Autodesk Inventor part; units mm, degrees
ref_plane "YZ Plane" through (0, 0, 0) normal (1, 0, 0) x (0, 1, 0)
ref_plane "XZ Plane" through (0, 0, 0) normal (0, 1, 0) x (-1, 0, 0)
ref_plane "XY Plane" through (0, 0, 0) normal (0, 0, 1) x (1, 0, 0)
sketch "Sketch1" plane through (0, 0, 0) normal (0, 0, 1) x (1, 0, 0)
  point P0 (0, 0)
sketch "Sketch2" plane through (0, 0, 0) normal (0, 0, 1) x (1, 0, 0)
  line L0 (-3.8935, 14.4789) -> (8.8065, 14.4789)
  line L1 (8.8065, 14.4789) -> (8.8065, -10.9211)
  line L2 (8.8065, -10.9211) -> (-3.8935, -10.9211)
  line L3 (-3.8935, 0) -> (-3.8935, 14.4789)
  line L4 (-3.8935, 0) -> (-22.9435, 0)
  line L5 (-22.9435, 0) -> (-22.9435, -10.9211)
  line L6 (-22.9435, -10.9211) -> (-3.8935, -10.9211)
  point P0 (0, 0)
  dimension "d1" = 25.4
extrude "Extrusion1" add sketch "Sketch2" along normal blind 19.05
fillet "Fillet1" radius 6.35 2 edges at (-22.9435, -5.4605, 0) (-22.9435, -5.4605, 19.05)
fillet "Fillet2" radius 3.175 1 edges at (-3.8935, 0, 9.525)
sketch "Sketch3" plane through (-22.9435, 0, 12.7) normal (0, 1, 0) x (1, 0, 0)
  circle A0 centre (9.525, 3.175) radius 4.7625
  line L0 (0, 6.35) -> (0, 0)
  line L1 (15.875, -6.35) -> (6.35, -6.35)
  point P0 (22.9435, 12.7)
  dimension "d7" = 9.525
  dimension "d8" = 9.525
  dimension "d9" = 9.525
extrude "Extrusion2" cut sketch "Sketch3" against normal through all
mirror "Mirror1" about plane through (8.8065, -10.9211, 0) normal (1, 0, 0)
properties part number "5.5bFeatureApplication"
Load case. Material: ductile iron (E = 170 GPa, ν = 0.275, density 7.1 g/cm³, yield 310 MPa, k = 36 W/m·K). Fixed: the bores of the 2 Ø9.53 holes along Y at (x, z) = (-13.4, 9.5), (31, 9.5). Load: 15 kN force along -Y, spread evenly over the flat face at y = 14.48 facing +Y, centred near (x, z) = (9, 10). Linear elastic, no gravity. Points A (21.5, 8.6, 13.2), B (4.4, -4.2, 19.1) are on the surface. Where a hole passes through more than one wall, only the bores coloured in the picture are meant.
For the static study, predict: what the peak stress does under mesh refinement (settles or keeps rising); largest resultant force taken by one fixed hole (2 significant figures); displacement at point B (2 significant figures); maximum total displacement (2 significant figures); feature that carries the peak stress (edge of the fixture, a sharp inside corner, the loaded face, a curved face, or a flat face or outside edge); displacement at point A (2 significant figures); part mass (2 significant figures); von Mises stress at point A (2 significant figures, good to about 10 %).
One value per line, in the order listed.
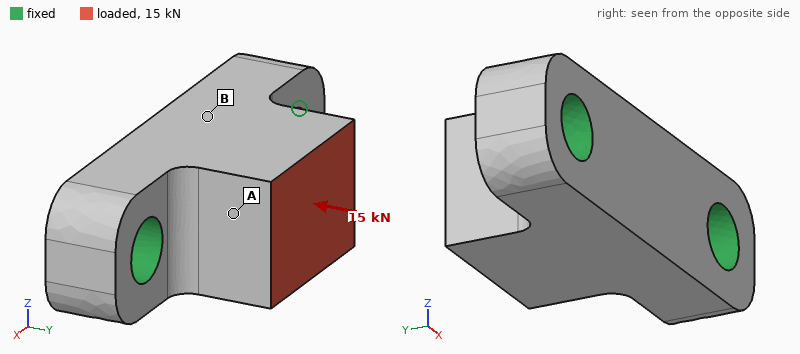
keeps rising
8.0 kN
8.9 µm
11 µm
edge of the fixture
9.4 µm
130 g
37 MPa
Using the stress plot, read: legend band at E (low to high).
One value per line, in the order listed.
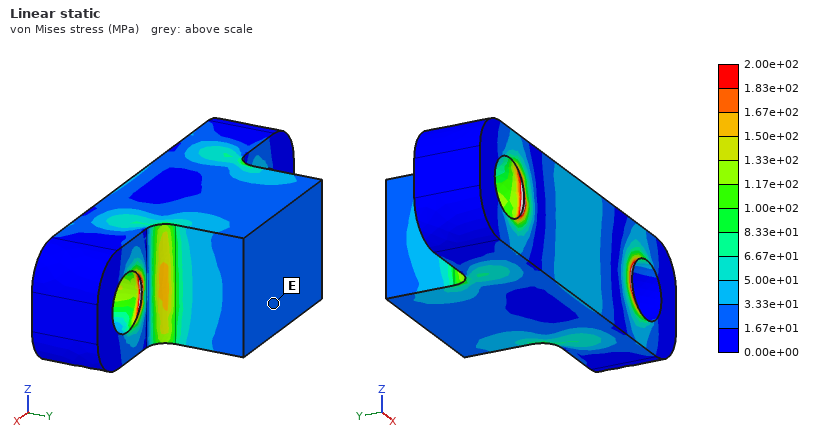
1.67e+01 to 3.33e+01 MPa
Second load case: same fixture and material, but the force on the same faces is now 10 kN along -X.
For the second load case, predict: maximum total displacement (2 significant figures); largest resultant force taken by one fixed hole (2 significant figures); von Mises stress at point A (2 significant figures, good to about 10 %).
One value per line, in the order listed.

17 µm
7.6 kN
39 MPa
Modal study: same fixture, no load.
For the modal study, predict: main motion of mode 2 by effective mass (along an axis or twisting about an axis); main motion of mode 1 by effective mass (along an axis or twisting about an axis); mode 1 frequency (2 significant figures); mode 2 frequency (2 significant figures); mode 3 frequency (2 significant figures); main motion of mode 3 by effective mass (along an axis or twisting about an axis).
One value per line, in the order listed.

along Y
along Z
12 kHz
22 kHz
27 kHz
along X
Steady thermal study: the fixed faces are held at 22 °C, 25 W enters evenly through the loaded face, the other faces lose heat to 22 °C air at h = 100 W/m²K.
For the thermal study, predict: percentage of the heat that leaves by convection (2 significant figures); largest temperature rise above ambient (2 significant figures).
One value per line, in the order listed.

19 %
36 K
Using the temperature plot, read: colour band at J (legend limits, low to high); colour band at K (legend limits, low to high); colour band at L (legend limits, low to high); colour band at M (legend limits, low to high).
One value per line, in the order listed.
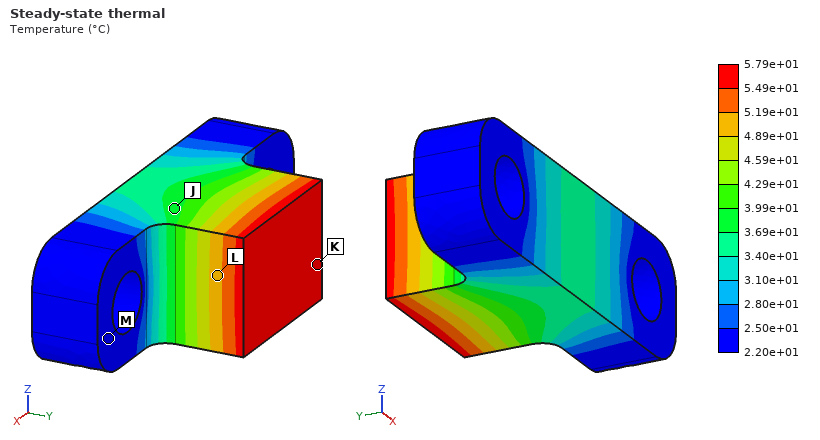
3.69e+01 to 3.99e+01 °C
5.49e+01 to 5.79e+01 °C
4.89e+01 to 5.19e+01 °C
2.20e+01 to 2.50e+01 °C
